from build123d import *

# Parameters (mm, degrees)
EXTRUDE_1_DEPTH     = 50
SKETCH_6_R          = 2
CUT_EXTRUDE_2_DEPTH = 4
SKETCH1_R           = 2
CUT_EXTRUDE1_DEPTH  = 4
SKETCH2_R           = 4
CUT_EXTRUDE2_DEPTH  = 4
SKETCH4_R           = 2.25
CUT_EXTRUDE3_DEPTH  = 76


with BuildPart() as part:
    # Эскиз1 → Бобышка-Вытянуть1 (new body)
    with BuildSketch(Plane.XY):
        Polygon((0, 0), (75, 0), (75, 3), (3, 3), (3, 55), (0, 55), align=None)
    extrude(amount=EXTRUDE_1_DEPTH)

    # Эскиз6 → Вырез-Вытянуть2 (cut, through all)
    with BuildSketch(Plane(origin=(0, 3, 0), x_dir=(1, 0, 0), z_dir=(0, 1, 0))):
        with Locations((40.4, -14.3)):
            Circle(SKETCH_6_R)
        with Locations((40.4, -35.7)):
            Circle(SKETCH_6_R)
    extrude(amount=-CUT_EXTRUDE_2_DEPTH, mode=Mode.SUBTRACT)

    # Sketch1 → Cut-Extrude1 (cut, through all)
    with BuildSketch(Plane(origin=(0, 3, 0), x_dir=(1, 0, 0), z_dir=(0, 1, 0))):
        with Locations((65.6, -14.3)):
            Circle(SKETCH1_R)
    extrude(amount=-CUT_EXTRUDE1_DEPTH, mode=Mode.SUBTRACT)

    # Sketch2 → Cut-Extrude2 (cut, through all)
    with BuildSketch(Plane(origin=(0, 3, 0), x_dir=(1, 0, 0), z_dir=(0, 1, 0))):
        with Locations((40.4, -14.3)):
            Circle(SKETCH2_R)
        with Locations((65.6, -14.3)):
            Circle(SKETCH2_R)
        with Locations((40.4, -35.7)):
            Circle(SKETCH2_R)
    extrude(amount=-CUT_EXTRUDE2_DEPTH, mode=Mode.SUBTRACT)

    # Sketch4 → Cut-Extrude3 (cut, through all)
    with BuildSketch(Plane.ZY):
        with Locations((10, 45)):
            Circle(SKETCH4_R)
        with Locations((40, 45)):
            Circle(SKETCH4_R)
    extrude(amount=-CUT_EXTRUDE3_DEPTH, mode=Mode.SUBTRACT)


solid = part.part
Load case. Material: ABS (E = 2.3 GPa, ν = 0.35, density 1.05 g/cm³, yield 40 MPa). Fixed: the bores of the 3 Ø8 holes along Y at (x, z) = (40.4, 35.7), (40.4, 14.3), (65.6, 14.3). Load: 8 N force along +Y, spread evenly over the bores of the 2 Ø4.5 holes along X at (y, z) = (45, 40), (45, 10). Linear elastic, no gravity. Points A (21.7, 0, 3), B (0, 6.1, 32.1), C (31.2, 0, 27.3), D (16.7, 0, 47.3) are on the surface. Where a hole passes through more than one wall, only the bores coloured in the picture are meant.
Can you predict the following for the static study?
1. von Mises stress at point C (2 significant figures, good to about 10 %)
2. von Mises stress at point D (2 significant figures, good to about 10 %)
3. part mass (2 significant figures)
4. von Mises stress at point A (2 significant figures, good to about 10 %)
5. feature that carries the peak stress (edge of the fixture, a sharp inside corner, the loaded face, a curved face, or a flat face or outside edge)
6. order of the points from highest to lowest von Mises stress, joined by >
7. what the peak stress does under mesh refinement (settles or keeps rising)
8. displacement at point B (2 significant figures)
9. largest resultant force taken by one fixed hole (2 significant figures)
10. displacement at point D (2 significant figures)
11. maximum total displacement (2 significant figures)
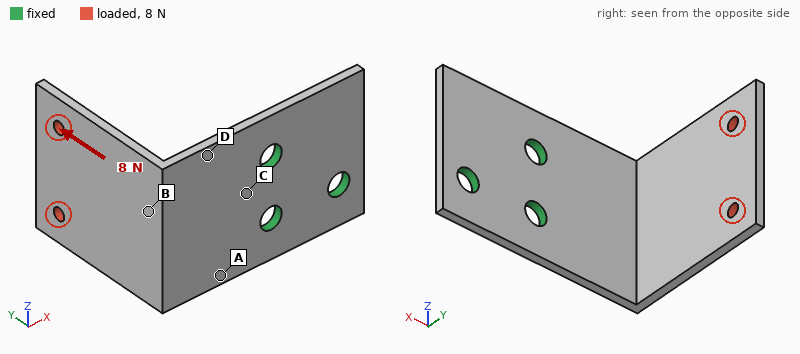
2.8 MPa
1.6 MPa
19 g
2.1 MPa
edge of the fixture
C > A > D > B
keeps rising
0.50 mm
4.4 N
0.19 mm
1.1 mm
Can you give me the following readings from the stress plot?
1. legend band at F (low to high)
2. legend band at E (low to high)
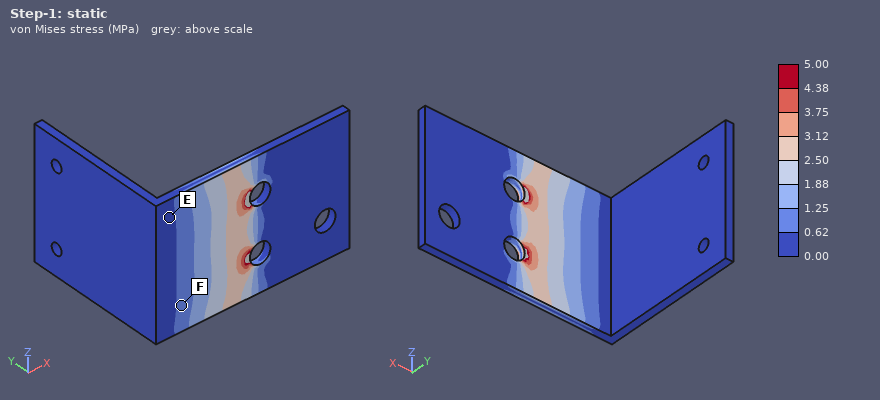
0.62 to 1.25 MPa
0.00 to 0.62 MPa
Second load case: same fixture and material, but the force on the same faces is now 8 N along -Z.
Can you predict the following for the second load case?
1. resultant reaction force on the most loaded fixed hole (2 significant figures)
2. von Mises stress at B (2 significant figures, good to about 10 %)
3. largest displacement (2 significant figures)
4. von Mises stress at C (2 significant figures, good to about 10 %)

15 N
1.4 MPa
1.2 mm
1.7 MPa
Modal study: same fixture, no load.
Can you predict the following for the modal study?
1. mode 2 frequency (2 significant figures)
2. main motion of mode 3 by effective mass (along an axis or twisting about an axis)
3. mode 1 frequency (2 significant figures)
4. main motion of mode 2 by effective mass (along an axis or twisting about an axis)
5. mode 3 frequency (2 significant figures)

210 Hz
along Y
120 Hz
along Z
350 Hz
